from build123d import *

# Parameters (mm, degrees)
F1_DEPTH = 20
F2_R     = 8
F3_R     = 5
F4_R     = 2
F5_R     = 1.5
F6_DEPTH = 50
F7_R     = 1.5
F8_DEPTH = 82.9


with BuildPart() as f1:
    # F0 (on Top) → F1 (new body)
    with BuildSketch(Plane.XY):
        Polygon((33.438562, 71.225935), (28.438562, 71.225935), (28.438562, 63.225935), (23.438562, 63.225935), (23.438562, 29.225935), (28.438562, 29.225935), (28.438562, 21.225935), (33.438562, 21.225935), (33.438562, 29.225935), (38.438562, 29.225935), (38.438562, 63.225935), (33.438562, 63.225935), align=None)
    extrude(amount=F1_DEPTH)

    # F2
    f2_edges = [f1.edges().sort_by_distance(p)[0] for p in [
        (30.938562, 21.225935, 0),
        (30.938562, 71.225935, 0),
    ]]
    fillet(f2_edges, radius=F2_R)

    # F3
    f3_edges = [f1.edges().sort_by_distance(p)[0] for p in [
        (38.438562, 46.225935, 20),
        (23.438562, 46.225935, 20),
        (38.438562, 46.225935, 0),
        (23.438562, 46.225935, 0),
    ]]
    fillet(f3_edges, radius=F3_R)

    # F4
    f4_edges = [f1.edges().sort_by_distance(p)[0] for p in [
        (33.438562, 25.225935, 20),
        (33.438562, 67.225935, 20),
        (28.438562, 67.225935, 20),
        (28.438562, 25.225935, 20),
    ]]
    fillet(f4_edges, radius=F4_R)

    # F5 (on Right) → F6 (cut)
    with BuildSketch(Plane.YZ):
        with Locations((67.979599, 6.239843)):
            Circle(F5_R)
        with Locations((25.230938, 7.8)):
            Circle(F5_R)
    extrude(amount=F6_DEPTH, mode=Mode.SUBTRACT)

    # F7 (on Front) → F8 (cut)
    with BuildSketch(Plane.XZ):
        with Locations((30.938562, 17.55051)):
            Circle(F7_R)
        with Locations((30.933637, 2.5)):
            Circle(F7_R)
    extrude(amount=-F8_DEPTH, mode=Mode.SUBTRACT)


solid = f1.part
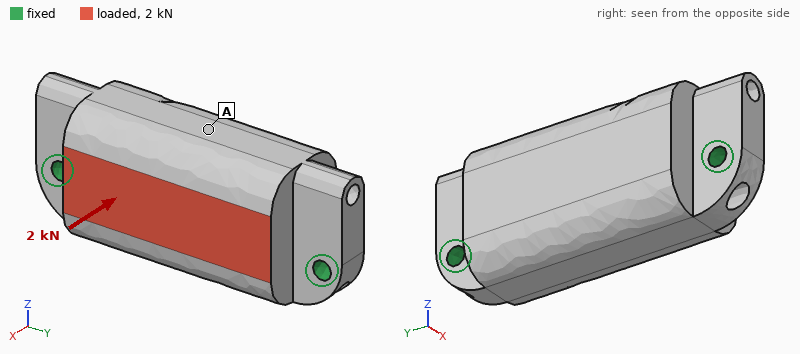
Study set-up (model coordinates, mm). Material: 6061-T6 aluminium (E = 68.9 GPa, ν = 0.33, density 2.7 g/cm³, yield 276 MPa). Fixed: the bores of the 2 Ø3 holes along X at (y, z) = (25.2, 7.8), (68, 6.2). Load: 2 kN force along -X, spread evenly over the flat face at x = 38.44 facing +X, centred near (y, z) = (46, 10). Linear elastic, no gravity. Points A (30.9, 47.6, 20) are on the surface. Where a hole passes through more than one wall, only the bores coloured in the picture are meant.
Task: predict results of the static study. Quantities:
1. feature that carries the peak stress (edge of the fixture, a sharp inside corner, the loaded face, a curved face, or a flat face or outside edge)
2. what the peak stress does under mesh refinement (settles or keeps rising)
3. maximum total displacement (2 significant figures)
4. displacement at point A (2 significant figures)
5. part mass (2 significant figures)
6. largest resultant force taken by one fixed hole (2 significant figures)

edge of the fixture
keeps rising
25 µm
25 µm
27 g
1.0 kN
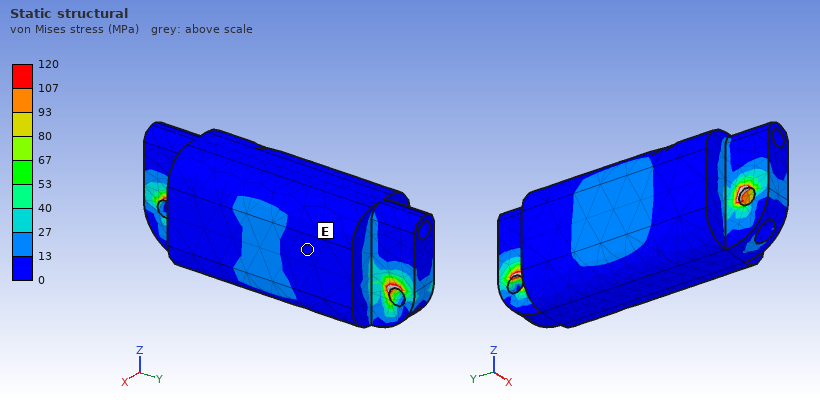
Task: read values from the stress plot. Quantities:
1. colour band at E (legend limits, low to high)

0 to 13 MPa
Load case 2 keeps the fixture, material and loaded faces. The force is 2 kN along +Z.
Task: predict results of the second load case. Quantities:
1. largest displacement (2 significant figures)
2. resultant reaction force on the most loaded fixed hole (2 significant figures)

50 µm
1.1 kN
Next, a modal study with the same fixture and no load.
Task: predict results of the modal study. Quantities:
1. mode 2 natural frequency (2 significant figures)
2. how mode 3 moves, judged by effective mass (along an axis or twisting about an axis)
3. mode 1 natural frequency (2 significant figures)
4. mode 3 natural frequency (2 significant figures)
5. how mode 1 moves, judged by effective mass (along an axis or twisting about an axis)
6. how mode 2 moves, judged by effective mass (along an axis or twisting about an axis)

15 kHz
along Z
8800 Hz
17 kHz
along X
along X
